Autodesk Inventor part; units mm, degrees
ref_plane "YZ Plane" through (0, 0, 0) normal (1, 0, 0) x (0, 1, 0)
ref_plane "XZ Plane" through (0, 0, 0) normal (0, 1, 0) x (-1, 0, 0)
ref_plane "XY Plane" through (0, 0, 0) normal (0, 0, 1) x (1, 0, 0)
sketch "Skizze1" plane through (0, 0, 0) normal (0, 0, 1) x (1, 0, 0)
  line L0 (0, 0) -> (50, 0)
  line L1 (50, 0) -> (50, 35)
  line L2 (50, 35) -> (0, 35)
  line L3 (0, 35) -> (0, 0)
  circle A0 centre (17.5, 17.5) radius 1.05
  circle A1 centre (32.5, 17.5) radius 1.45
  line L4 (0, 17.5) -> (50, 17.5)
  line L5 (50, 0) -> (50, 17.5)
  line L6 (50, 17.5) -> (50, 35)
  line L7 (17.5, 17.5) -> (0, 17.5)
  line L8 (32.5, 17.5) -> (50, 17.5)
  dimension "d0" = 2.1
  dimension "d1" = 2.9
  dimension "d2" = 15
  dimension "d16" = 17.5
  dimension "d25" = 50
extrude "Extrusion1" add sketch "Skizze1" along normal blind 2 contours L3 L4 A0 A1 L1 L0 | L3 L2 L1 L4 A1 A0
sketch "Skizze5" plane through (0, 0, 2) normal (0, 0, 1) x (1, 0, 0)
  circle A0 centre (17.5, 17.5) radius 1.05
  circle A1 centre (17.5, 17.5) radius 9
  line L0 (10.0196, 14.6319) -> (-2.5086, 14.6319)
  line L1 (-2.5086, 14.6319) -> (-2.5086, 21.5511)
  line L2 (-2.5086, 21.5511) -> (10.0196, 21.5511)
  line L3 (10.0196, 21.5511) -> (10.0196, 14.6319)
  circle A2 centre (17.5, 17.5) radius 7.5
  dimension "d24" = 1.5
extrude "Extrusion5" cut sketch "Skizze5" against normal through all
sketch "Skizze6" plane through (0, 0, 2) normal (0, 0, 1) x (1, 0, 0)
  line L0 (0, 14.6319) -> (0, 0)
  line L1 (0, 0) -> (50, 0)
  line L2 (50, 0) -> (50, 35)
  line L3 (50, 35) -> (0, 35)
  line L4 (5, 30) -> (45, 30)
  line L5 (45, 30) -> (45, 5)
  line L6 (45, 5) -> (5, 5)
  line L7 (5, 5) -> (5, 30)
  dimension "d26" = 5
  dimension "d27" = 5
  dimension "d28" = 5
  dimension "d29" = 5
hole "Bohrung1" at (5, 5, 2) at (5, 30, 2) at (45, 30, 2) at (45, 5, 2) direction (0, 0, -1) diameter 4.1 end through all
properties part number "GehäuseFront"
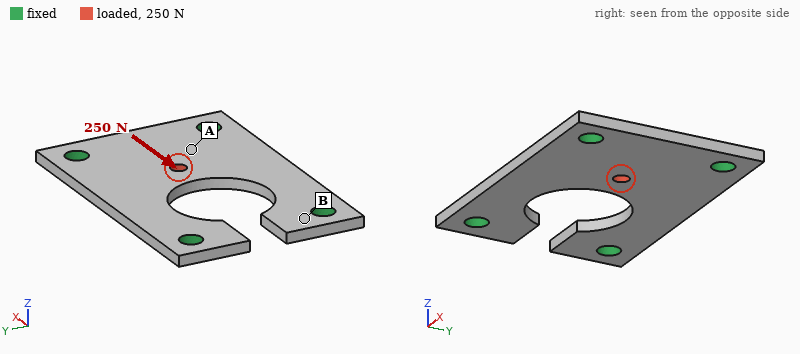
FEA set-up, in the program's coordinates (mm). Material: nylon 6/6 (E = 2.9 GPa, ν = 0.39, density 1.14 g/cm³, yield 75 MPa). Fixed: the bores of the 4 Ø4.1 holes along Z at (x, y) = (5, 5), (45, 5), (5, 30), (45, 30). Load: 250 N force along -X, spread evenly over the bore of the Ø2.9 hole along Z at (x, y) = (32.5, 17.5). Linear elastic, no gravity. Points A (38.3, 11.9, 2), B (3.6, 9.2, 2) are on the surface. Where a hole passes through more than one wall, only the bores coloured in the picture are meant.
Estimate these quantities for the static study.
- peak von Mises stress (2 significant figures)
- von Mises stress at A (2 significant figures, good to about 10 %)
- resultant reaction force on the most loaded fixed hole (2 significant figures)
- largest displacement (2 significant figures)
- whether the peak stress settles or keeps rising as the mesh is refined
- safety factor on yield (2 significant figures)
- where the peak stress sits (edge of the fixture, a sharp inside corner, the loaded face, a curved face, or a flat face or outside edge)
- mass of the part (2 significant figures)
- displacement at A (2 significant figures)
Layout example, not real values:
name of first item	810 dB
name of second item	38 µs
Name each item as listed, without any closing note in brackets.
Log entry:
peak von Mises stress	25 MPa
von Mises stress at A	6.4 MPa
resultant reaction force on the most loaded fixed hole	110 N
largest displacement	58 µm
whether the peak stress settles or keeps rising as the mesh is refined	settles
safety factor on yield	3.0
where the peak stress sits	the loaded face
mass of the part	3.1 g
displacement at A	24 µm
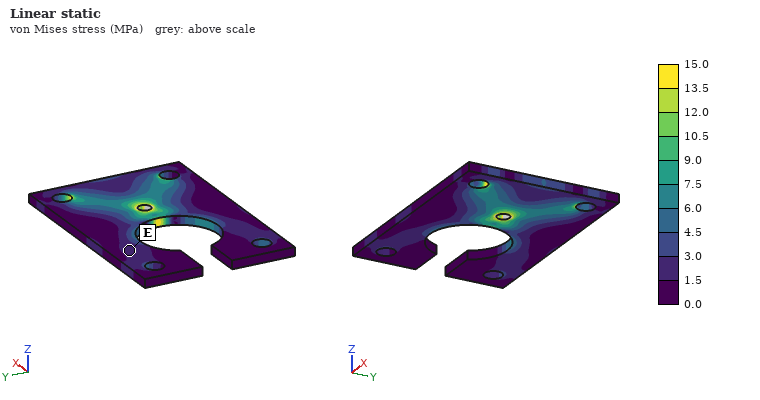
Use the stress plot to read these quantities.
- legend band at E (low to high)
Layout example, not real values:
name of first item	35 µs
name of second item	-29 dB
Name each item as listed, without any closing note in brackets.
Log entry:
legend band at E	1.5 to 3.0 MPa
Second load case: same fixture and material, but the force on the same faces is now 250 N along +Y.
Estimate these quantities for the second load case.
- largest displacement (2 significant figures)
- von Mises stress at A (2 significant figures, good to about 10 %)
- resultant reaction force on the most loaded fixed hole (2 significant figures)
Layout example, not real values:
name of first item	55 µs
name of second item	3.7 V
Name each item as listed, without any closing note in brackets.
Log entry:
largest displacement	63 µm
von Mises stress at A	7.3 MPa
resultant reaction force on the most loaded fixed hole	130 N
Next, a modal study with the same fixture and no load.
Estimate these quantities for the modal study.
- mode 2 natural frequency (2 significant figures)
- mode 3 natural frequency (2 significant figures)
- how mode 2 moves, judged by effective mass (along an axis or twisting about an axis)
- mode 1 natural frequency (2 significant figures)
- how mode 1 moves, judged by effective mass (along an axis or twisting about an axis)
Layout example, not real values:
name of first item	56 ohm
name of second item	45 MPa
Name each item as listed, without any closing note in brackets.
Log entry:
mode 2 natural frequency	2700 Hz
mode 3 natural frequency	4100 Hz
how mode 2 moves, judged by effective mass	twisting about X
mode 1 natural frequency	2200 Hz
how mode 1 moves, judged by effective mass	along Z
